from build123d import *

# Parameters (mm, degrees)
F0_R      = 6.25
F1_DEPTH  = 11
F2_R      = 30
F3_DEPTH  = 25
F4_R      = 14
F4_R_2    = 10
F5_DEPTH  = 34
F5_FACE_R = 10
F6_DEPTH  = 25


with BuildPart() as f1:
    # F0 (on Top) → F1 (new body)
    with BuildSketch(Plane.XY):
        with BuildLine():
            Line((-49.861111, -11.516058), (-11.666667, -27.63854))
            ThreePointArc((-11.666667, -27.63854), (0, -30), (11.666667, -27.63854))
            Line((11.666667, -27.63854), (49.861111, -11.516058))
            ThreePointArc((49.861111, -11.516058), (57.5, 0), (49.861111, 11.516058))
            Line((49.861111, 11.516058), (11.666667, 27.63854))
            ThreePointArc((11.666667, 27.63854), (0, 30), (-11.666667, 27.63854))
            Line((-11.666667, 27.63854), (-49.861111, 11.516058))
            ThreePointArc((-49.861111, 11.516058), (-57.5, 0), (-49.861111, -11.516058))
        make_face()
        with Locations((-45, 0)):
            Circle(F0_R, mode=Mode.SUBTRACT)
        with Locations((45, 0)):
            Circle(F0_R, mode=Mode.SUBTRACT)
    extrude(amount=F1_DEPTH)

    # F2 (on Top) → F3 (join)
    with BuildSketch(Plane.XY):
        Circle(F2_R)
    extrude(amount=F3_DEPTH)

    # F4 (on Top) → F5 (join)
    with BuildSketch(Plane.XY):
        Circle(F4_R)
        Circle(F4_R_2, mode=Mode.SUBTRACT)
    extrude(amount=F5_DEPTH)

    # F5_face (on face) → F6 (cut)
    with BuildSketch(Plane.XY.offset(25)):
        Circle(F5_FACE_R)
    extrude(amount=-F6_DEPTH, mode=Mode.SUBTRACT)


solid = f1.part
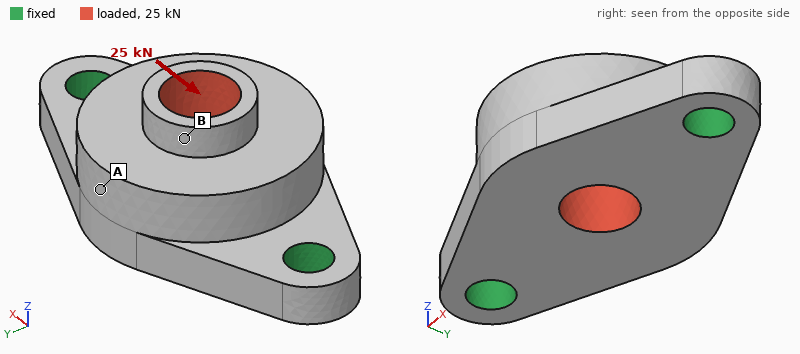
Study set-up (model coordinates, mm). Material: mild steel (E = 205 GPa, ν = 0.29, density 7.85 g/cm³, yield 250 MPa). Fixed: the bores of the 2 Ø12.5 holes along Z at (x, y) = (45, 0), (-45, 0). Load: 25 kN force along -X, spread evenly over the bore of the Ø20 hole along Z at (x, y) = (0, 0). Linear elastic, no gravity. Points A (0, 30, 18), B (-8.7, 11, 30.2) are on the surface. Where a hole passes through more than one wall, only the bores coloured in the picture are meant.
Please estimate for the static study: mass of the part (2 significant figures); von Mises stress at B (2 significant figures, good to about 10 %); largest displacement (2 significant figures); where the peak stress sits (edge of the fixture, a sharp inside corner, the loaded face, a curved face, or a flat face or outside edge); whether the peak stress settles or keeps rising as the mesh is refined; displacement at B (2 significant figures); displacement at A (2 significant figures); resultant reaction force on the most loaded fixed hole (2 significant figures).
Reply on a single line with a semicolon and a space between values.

650 g; 19 MPa; 14 µm; edge of the fixture; keeps rising; 11 µm; 5.4 µm; 13 kN
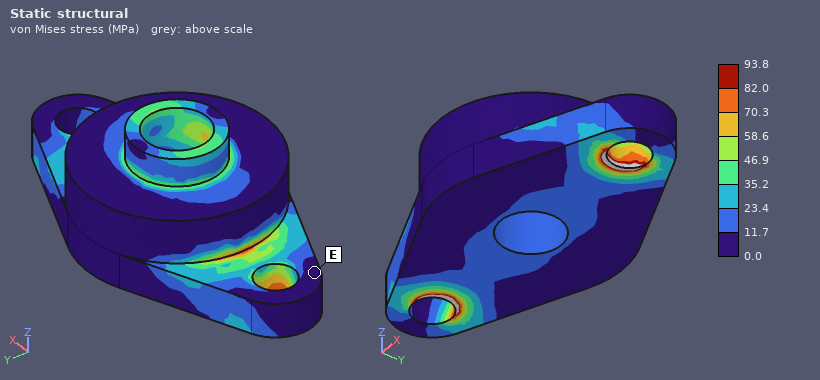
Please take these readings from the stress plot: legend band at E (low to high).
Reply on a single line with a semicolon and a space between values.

0.0 to 11.7 MPa
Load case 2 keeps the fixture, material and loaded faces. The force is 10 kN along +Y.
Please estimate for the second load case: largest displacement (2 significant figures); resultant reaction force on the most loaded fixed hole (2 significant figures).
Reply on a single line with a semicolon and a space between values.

32 µm; 5.0 kN
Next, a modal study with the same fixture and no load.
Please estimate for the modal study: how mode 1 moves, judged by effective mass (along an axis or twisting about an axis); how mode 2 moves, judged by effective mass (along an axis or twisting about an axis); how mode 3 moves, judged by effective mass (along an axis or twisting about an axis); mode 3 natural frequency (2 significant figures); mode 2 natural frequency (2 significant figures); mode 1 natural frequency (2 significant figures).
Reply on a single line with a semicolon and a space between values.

along Y; along Z; along Y; 11 kHz; 6900 Hz; 4300 Hz
